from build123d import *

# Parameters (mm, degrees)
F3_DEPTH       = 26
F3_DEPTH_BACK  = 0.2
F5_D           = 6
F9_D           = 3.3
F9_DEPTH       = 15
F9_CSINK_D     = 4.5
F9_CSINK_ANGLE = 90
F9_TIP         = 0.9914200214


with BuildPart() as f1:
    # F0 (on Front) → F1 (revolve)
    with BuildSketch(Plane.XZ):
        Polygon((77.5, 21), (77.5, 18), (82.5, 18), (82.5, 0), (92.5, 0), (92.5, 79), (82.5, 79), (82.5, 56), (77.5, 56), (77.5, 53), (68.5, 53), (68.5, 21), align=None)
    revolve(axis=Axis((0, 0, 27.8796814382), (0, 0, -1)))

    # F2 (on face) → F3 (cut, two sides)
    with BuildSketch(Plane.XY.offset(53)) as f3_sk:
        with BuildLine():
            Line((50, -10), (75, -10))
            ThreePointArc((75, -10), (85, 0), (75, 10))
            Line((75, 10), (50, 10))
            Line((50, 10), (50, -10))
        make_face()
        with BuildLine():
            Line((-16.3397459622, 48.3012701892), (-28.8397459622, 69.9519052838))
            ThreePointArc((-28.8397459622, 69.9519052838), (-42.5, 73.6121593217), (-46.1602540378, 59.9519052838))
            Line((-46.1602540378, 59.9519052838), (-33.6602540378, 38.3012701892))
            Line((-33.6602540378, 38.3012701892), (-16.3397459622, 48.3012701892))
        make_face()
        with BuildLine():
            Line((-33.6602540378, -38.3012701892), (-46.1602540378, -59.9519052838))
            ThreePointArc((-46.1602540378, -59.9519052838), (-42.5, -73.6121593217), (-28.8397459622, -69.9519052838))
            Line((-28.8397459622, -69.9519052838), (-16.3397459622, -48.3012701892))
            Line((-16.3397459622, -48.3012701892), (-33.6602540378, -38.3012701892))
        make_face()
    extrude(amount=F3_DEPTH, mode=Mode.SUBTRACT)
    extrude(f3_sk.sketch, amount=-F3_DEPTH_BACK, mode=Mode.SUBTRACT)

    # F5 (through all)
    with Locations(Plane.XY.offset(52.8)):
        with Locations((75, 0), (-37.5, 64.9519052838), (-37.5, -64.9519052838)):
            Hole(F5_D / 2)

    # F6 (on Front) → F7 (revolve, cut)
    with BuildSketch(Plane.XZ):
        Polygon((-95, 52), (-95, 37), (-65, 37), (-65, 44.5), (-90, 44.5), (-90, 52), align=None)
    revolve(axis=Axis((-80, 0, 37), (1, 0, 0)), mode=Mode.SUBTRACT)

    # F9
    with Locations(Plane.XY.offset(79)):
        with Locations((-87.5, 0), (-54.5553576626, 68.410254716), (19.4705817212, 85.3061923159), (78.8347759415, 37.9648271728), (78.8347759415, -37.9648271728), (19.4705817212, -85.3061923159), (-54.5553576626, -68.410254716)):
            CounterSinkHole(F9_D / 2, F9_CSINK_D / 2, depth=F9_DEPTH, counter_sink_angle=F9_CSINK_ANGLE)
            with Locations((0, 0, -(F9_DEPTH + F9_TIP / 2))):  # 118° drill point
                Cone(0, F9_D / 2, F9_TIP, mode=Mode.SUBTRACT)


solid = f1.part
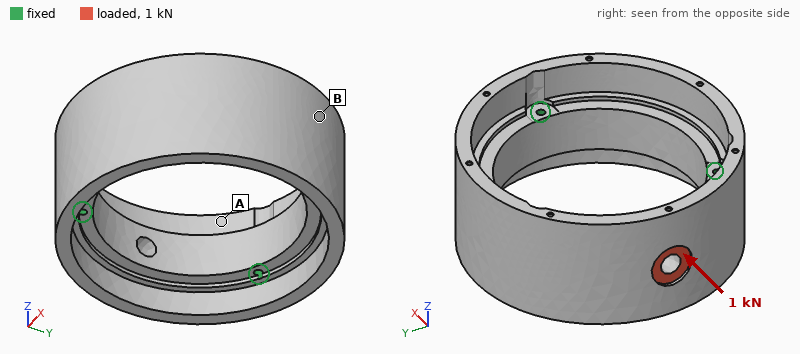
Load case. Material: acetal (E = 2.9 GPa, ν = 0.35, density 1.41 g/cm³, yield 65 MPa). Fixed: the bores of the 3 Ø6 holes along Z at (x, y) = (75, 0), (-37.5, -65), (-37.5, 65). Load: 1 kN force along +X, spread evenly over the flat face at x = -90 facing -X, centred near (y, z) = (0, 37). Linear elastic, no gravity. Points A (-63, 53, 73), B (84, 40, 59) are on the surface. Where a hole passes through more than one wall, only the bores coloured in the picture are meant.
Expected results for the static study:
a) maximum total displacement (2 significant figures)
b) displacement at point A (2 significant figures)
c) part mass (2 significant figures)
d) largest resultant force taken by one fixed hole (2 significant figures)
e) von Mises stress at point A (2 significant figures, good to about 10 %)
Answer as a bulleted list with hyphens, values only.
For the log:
- 72 µm
- 14 µm
- 920 g
- 740 N
- 0.60 MPa
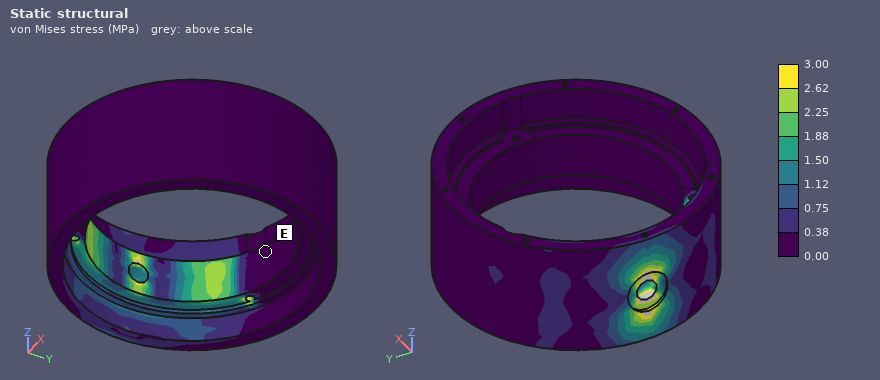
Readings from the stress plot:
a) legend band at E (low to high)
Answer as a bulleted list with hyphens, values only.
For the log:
- 0.00 to 0.38 MPa
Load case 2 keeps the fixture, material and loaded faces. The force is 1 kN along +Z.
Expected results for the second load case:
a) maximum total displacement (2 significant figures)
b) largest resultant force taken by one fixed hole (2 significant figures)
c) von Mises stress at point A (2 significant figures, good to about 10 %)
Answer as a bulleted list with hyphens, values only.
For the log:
- 0.25 mm
- 580 N
- 1.6 MPa
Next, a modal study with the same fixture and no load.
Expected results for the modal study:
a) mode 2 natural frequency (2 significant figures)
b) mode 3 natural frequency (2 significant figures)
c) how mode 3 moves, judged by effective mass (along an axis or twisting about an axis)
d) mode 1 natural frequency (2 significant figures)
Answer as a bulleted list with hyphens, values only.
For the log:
- 950 Hz
- 1300 Hz
- twisting about Z
- 940 Hz
